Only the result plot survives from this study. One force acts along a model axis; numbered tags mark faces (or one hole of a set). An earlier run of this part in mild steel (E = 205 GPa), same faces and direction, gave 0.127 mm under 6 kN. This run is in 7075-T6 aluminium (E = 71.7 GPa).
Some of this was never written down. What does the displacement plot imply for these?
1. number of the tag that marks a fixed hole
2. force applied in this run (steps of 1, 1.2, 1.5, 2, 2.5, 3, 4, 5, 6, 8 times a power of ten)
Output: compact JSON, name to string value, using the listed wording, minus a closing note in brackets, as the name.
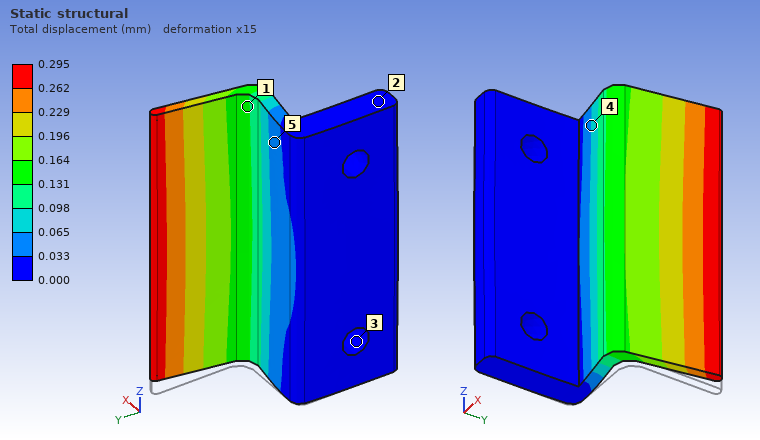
{"number of the tag that marks a fixed hole": "3", "force applied in this run": "5 kN"}
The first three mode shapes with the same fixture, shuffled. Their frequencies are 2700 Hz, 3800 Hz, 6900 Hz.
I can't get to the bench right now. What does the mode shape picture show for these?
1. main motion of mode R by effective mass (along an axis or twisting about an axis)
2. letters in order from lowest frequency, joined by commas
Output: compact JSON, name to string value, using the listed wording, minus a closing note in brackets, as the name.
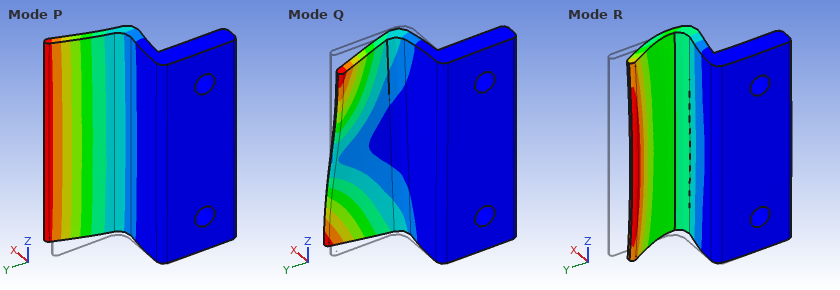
{"main motion of mode R by effective mass": "along Y", "letters in order from lowest frequency, joined by commas": "P, Q, R"}
